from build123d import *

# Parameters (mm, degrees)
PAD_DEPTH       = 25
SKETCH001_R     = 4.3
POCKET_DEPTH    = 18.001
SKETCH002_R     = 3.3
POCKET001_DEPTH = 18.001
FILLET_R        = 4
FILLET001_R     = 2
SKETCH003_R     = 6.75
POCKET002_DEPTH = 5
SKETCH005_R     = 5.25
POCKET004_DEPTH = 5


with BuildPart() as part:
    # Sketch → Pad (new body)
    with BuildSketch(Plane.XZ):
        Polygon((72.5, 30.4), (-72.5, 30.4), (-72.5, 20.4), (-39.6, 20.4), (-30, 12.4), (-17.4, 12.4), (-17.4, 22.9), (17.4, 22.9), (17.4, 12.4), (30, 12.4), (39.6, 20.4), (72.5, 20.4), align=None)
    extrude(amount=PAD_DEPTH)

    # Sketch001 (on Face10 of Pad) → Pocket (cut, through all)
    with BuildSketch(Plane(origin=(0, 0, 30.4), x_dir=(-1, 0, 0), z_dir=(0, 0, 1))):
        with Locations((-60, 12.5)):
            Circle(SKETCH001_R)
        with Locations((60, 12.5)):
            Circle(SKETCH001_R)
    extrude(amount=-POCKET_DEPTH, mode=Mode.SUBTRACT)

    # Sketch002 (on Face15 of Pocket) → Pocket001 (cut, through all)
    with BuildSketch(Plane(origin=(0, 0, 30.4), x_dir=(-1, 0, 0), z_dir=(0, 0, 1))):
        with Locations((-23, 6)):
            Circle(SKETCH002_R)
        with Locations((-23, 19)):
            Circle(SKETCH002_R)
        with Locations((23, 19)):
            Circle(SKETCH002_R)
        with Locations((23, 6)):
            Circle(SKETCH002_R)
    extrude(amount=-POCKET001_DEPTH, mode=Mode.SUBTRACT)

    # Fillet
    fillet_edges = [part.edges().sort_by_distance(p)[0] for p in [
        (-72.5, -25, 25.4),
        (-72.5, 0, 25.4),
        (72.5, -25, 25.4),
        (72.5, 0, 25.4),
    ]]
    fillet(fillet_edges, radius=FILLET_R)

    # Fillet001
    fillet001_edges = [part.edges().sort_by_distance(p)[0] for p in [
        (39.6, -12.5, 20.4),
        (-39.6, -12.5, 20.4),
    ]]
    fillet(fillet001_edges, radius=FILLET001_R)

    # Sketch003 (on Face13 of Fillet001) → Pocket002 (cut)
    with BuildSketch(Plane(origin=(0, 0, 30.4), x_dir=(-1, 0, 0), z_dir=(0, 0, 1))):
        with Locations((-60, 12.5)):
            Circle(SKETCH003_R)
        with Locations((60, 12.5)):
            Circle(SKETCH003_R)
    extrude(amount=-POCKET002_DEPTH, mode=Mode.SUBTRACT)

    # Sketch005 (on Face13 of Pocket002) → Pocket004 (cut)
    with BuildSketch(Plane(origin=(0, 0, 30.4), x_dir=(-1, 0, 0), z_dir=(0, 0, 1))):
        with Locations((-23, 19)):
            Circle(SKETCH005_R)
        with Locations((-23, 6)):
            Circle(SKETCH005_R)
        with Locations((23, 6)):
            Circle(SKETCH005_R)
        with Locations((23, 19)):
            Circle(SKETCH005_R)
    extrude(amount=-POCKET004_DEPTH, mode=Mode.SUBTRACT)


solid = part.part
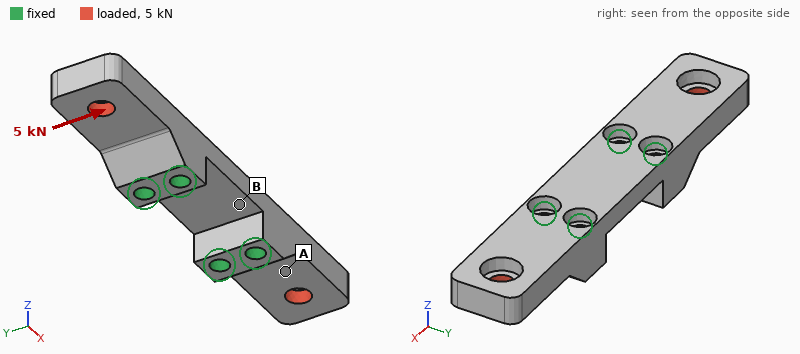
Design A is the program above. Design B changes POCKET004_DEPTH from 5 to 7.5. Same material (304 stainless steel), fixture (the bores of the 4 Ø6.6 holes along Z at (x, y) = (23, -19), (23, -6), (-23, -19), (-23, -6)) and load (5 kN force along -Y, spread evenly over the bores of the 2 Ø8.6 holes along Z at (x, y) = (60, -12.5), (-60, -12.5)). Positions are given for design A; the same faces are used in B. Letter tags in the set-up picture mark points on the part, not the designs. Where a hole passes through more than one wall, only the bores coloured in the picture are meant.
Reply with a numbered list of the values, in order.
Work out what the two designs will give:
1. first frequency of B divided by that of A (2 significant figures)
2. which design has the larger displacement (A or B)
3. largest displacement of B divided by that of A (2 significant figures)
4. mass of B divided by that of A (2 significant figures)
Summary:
1. 0.92
2. B
3. 1.1
4. 0.99
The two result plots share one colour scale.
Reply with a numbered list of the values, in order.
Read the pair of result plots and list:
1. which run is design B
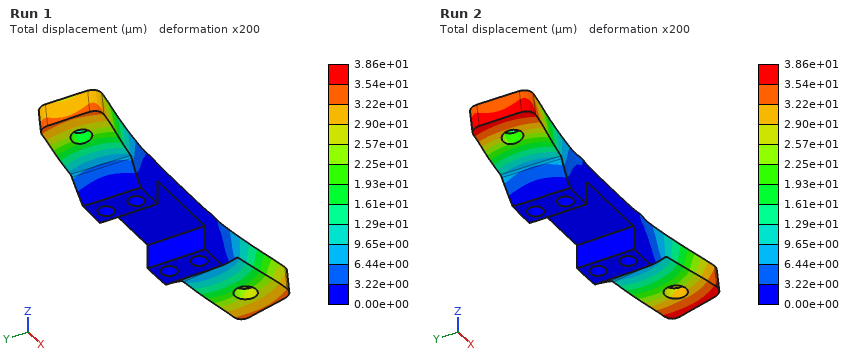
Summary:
1. Run 2
